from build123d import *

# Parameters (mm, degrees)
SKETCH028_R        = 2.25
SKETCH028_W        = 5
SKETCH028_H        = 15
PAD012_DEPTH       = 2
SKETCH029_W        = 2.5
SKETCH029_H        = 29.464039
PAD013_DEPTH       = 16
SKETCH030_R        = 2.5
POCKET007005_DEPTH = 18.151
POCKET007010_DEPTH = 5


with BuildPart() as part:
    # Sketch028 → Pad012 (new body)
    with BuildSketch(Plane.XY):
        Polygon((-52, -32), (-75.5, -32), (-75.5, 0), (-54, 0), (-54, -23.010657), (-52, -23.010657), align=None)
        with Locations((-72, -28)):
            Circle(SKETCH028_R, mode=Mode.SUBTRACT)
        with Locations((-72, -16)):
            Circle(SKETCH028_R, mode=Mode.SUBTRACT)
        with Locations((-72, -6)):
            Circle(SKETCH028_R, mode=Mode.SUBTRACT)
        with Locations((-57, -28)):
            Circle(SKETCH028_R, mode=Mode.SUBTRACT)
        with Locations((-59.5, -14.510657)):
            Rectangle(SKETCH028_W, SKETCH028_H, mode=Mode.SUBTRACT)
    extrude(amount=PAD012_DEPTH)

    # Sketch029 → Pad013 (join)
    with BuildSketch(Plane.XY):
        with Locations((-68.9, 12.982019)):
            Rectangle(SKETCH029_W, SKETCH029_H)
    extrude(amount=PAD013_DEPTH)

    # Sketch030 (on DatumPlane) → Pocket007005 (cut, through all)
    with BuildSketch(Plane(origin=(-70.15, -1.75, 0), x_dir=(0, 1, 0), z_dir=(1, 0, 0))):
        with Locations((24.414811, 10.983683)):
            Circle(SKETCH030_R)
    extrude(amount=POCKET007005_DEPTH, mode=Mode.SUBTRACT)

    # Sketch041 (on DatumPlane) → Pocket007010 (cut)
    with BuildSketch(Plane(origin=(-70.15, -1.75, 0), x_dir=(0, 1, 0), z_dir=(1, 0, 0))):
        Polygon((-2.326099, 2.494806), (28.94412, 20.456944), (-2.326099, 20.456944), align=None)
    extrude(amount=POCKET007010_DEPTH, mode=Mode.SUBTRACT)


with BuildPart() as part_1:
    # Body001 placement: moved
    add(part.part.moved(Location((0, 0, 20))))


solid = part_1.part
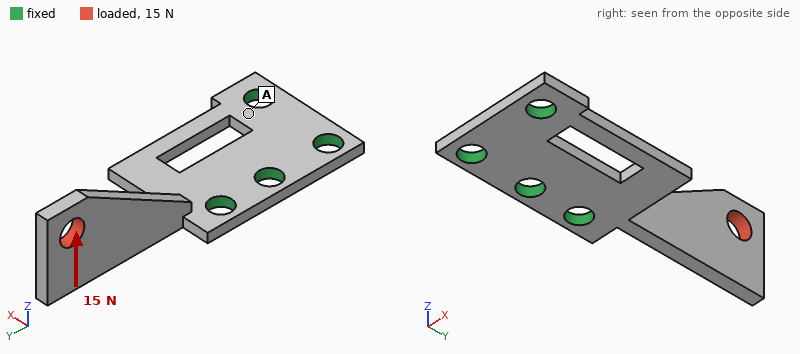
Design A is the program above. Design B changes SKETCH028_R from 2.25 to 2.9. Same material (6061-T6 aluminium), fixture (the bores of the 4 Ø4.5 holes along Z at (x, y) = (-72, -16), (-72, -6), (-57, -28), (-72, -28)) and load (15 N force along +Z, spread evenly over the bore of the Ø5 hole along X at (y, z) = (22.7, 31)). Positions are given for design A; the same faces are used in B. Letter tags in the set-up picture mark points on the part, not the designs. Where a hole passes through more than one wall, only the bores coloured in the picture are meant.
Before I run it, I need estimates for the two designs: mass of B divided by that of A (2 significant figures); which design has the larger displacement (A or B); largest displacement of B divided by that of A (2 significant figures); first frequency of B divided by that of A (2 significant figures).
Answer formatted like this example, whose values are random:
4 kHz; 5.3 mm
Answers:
0.96; A; 0.90; 1.0
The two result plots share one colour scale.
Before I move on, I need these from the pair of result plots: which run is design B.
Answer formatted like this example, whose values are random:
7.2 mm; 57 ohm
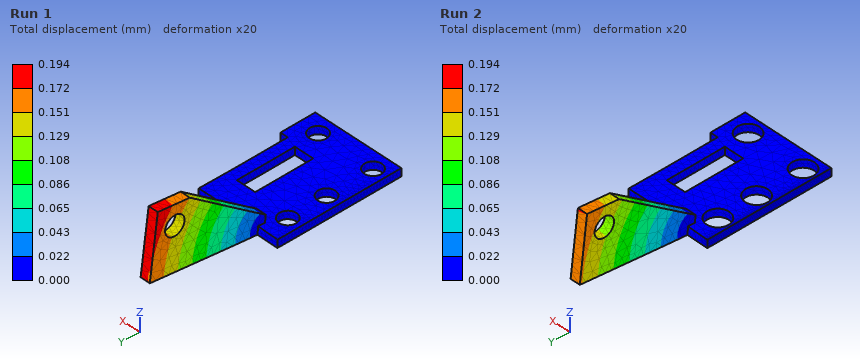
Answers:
Run 2
